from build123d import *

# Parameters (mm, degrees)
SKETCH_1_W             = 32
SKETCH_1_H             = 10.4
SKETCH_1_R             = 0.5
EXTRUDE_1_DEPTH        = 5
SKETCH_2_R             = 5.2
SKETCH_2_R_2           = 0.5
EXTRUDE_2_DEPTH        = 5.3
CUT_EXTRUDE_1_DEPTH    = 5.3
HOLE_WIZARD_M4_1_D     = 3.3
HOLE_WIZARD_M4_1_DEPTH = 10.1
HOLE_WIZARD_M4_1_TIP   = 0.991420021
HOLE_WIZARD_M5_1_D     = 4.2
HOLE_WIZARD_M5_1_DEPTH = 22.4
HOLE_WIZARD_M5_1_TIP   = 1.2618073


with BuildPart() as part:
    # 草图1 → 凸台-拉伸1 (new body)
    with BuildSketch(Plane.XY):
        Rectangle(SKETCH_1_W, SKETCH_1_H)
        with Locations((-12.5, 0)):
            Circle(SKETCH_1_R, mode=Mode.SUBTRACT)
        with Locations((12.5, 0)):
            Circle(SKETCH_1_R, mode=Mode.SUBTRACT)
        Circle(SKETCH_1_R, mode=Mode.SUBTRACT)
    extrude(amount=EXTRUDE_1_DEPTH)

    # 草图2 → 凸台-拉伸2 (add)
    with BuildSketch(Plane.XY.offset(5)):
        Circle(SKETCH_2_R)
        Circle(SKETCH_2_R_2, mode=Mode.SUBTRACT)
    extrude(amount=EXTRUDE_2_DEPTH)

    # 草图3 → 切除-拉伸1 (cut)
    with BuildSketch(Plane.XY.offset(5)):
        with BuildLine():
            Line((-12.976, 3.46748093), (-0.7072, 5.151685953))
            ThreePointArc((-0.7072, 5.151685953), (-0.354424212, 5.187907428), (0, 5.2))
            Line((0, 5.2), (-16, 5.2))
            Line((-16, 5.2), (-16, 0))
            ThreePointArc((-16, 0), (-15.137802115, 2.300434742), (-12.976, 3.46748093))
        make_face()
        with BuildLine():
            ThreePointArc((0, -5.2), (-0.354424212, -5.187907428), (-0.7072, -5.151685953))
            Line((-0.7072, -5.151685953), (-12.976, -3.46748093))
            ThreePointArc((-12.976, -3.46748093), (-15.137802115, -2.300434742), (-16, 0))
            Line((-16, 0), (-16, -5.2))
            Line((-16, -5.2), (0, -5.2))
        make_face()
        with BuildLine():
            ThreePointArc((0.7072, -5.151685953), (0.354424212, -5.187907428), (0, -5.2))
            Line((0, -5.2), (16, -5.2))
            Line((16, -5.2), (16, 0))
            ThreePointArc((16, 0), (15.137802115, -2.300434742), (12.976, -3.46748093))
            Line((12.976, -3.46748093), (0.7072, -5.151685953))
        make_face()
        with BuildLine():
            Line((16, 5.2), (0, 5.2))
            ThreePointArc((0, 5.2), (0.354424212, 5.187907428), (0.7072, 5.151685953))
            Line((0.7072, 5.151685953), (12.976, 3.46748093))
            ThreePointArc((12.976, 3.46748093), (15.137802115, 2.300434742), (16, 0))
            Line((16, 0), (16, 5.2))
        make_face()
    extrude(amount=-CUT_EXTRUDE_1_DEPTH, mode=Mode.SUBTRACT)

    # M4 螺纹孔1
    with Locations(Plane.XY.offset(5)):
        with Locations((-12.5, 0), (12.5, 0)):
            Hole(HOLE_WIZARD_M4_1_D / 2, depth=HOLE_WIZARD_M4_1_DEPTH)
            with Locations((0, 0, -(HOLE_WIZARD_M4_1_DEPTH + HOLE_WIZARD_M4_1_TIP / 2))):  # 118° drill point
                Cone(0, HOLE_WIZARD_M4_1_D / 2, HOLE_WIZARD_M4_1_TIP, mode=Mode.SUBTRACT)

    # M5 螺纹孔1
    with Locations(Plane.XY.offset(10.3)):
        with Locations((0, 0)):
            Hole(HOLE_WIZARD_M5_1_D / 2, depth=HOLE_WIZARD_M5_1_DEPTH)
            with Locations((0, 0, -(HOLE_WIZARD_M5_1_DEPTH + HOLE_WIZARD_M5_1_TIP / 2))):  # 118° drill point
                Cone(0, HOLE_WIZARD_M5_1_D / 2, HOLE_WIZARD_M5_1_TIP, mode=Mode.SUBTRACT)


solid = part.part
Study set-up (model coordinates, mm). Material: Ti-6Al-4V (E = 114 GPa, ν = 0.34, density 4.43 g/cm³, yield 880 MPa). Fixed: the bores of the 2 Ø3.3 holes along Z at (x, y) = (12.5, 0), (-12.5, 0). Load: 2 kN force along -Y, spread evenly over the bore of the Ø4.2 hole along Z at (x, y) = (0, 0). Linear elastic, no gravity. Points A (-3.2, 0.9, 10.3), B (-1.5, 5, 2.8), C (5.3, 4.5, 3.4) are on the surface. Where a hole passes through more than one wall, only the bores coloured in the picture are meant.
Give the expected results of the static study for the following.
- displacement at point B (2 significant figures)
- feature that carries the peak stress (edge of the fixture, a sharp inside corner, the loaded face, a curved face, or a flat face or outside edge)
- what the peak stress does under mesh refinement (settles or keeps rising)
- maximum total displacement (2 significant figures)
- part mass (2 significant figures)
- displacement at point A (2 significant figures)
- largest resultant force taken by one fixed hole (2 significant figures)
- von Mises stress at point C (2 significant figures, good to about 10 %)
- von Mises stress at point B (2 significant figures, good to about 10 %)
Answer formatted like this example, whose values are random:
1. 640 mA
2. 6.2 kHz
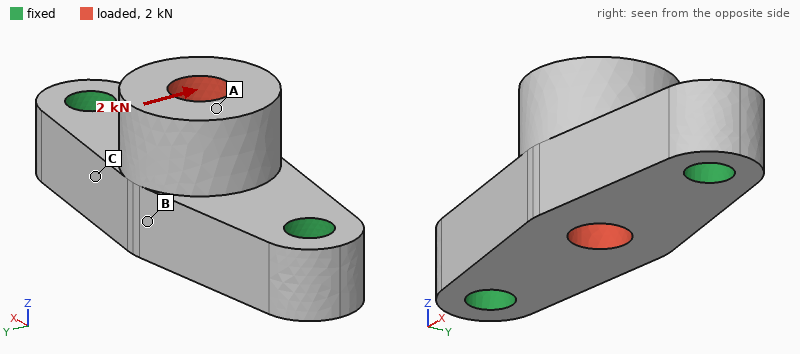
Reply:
1. 16 µm
2. edge of the fixture
3. keeps rising
4. 33 µm
5. 6.7 g
6. 30 µm
7. 1.0 kN
8. 88 MPa
9. 74 MPa
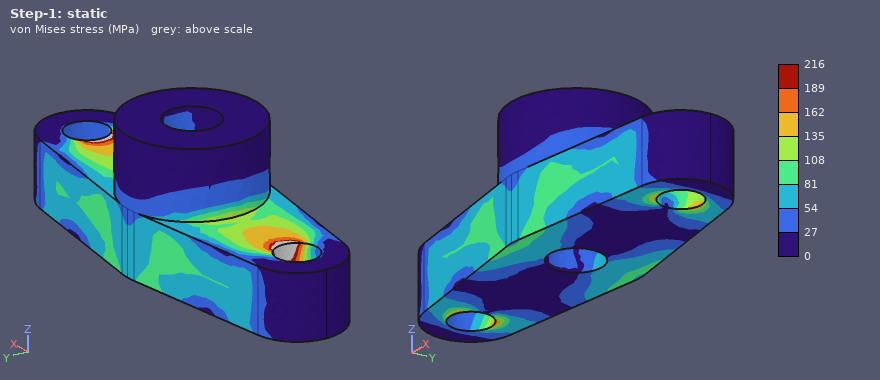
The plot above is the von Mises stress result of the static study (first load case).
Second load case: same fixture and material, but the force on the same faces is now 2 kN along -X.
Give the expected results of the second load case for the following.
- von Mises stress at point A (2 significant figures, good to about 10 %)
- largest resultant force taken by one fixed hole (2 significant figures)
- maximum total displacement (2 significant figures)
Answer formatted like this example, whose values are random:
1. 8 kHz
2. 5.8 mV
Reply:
1. 20 MPa
2. 1.0 kN
3. 6.7 µm
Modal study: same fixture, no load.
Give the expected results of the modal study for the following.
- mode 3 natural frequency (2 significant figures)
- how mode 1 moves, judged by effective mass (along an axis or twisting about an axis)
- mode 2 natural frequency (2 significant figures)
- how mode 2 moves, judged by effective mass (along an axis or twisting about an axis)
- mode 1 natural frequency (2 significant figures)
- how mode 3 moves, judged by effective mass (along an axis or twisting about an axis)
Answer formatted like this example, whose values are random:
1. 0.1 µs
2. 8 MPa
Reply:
1. 43 kHz
2. along Y
3. 31 kHz
4. along Z
5. 24 kHz
6. along Y
